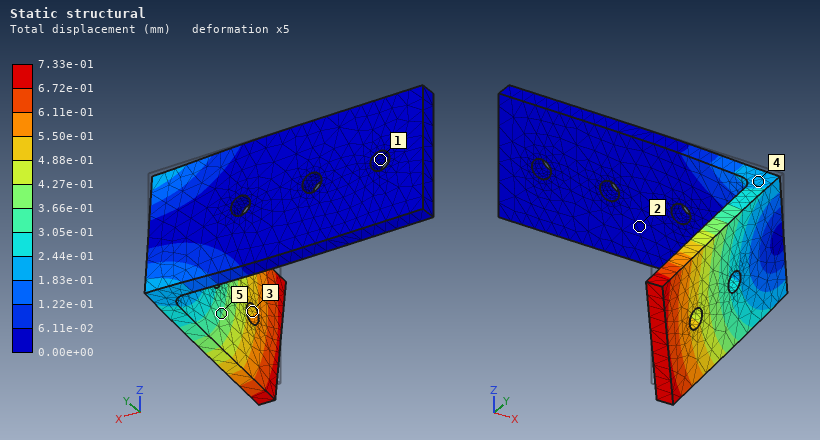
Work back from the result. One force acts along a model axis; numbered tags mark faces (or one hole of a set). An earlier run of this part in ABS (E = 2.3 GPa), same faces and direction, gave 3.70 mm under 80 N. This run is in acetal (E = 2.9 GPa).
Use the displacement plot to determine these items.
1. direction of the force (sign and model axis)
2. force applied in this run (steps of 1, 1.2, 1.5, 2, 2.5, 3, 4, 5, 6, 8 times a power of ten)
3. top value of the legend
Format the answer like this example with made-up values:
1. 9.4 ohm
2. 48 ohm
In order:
1. -Z
2. 20 N
3. 7.33e-01 mm
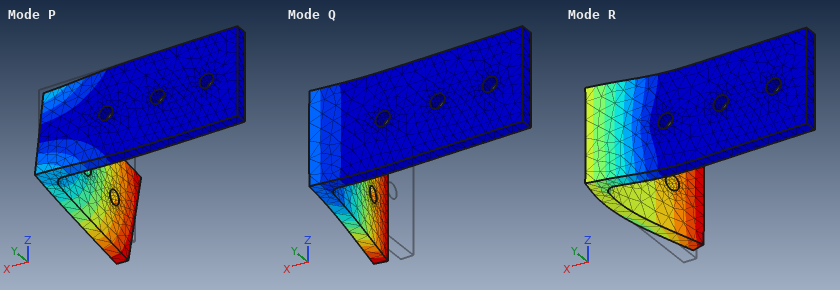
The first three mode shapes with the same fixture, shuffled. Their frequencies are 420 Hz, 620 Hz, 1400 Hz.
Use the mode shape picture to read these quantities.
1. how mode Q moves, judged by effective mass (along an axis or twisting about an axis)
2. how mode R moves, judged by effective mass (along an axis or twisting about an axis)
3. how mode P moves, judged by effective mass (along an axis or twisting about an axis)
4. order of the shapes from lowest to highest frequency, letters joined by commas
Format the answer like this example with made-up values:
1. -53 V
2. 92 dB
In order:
1. along X
2. along Y
3. along Z
4. Q, P, R
